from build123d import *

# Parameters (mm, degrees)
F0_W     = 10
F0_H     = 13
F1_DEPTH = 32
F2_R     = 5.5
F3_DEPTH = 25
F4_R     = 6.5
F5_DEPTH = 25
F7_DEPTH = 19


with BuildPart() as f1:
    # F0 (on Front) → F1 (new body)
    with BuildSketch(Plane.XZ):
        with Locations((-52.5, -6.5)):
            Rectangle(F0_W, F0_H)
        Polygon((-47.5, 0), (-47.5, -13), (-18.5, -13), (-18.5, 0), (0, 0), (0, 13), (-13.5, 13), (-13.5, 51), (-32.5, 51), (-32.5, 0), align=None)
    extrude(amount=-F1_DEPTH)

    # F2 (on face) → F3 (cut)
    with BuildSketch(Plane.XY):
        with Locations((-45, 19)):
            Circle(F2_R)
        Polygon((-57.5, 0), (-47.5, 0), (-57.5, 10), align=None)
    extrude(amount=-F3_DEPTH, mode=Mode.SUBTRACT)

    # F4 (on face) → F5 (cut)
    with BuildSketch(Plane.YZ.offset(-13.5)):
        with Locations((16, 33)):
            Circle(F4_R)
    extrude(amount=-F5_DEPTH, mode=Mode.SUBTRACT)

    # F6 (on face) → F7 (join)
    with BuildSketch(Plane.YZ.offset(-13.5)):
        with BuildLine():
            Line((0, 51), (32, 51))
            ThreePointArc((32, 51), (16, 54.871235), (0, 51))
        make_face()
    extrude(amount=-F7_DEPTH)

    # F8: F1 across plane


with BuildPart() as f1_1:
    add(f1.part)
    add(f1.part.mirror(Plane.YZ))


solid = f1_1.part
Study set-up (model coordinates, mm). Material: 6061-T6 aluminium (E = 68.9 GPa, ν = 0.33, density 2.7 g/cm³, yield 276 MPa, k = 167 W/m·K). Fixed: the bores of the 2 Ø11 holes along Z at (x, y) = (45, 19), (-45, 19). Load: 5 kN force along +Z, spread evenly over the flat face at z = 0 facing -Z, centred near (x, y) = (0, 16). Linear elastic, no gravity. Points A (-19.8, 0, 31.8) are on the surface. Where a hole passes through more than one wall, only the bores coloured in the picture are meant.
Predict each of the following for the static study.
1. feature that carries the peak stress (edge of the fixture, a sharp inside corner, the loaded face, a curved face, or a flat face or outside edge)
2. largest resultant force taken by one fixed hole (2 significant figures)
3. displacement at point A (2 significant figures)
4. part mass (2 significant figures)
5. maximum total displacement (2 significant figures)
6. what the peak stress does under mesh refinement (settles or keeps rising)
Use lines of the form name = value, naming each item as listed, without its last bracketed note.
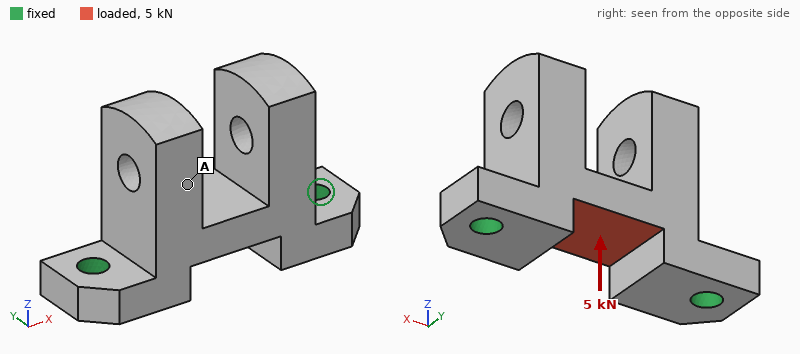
feature that carries the peak stress = edge of the fixture
largest resultant force taken by one fixed hole = 3.9 kN
displacement at point A = 22 µm
part mass = 270 g
maximum total displacement = 33 µm
what the peak stress does under mesh refinement = keeps rising
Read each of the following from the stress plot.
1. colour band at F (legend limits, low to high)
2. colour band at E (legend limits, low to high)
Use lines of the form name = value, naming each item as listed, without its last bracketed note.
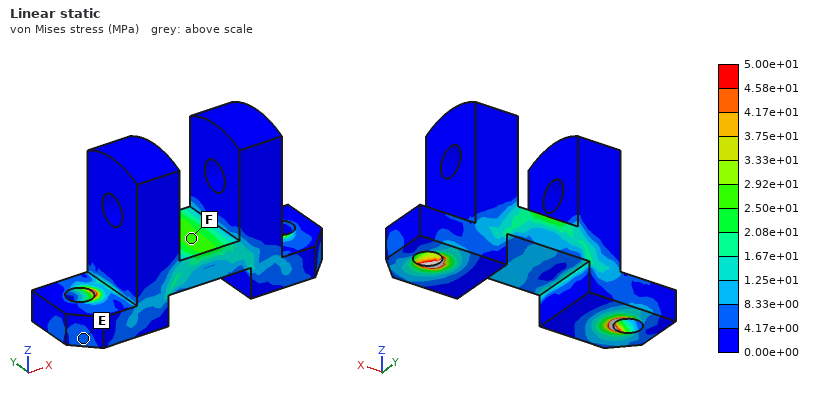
colour band at F = 2.50e+01 to 2.92e+01 MPa
colour band at E = 4.17e+00 to 8.33e+00 MPa
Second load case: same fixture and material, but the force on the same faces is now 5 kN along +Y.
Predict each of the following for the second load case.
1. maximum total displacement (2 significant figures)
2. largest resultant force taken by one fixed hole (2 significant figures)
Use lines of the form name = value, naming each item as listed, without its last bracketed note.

maximum total displacement = 39 µm
largest resultant force taken by one fixed hole = 2.5 kN
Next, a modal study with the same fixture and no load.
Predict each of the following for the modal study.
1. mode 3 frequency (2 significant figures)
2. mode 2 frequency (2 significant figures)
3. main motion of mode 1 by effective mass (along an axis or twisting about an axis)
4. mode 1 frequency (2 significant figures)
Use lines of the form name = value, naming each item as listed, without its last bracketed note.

mode 3 frequency = 4300 Hz
mode 2 frequency = 3900 Hz
main motion of mode 1 by effective mass = along Y
mode 1 frequency = 2500 Hz
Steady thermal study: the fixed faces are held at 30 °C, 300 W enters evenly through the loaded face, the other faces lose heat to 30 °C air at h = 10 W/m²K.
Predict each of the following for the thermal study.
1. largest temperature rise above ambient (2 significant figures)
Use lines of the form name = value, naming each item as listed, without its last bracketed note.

largest temperature rise above ambient = 79 K
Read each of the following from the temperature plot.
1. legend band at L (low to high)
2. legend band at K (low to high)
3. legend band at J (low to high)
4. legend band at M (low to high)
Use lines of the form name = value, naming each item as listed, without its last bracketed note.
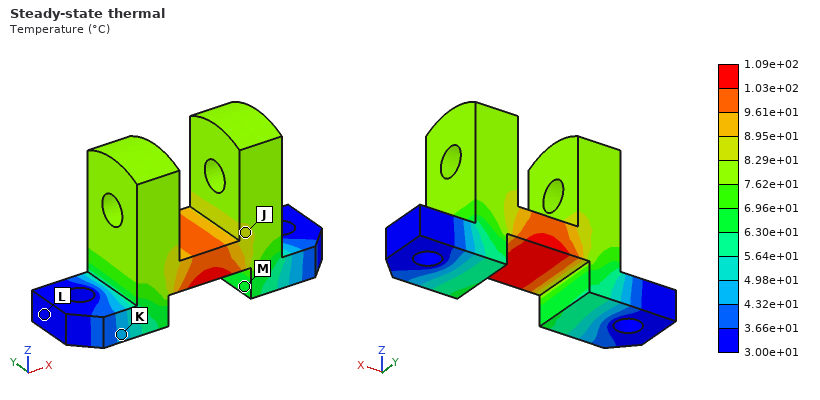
legend band at L = 3.00e+01 to 3.66e+01 °C
legend band at K = 4.32e+01 to 4.98e+01 °C
legend band at J = 8.29e+01 to 8.95e+01 °C
legend band at M = 6.30e+01 to 6.96e+01 °C
